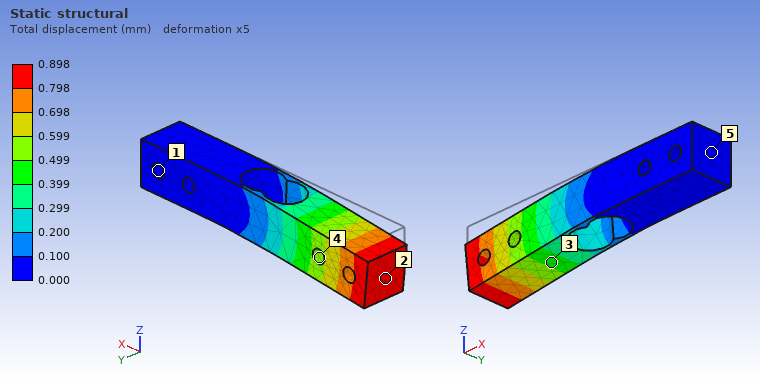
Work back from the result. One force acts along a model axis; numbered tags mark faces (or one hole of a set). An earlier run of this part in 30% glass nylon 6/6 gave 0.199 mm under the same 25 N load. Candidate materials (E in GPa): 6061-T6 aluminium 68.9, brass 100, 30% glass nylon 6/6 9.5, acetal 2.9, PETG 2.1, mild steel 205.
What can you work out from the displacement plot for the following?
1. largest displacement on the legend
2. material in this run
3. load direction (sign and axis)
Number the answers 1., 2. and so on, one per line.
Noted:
1. 0.898 mm
2. PETG
3. -Z
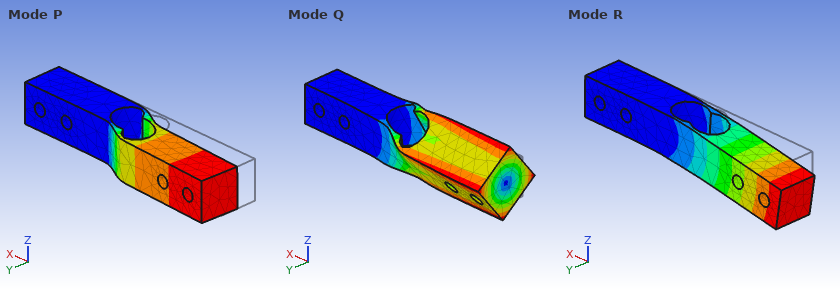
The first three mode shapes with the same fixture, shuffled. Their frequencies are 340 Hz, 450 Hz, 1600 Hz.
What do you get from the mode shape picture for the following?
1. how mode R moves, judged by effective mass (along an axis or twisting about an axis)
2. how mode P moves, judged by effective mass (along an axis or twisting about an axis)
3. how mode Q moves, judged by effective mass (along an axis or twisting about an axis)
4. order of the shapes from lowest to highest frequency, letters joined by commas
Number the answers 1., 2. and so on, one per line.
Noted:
1. along Z
2. along Y
3. twisting about X
4. P, R, Q
